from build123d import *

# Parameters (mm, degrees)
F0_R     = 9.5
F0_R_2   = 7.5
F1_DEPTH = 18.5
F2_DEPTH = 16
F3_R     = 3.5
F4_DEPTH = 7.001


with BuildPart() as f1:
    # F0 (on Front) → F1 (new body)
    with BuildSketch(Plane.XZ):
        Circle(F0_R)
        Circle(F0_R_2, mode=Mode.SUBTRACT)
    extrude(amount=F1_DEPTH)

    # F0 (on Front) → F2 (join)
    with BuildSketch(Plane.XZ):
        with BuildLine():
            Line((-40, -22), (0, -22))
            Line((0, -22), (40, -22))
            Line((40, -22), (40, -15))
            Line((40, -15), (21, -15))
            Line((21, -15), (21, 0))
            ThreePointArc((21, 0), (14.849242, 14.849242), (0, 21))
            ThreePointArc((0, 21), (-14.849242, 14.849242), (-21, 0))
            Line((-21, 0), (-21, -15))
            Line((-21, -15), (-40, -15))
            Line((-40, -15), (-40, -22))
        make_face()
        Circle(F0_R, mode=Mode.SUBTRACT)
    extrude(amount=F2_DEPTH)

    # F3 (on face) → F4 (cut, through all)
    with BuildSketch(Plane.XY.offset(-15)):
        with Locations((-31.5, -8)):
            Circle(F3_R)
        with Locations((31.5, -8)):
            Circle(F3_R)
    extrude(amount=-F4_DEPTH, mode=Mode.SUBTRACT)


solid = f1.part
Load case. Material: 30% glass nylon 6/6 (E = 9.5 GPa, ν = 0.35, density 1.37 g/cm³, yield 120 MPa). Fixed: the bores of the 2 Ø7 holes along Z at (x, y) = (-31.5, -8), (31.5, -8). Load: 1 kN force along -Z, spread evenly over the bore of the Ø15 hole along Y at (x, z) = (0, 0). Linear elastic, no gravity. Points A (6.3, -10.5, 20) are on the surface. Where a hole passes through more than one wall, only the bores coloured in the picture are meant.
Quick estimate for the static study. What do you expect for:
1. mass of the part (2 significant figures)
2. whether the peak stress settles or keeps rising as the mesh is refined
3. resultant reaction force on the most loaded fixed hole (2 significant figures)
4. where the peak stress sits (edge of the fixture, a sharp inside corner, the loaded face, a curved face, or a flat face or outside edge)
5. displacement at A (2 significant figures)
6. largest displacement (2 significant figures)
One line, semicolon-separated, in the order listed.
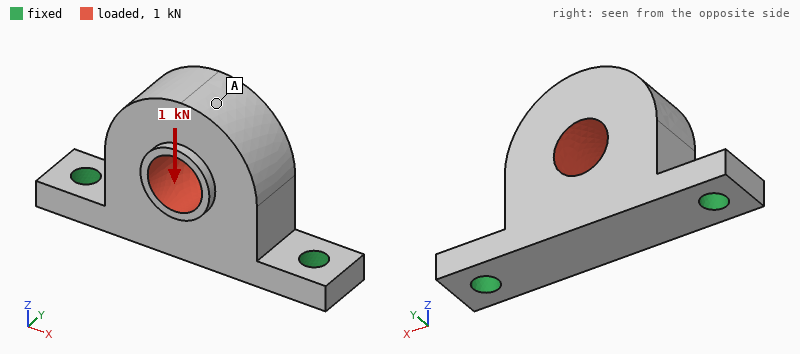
37 g; keeps rising; 560 N; edge of the fixture; 66 µm; 73 µm
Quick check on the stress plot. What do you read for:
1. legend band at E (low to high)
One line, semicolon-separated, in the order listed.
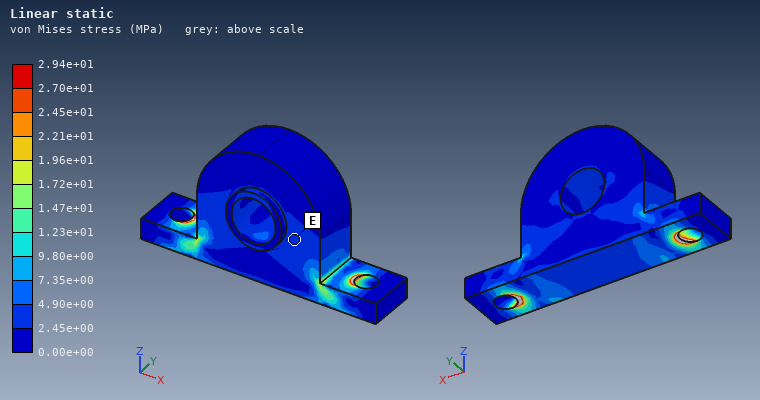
2.45e+00 to 4.90e+00 MPa
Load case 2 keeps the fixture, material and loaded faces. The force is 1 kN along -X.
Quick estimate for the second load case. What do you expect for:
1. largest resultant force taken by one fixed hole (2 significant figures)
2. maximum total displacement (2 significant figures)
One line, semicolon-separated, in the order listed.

620 N; 56 µm
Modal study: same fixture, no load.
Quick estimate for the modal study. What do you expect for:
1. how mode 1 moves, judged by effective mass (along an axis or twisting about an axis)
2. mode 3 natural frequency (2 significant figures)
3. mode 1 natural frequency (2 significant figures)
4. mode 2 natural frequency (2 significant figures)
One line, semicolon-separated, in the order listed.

along Y; 4600 Hz; 1300 Hz; 4500 Hz
